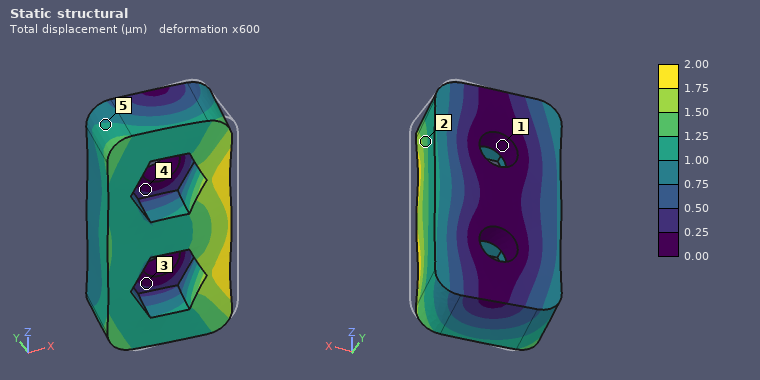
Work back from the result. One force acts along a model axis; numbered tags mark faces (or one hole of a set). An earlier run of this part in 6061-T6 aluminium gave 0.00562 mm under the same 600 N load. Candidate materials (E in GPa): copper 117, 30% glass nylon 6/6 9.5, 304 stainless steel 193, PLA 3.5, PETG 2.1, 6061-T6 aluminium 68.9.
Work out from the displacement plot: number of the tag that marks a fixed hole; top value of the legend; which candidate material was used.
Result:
1
2.00 µm
304 stainless steel
